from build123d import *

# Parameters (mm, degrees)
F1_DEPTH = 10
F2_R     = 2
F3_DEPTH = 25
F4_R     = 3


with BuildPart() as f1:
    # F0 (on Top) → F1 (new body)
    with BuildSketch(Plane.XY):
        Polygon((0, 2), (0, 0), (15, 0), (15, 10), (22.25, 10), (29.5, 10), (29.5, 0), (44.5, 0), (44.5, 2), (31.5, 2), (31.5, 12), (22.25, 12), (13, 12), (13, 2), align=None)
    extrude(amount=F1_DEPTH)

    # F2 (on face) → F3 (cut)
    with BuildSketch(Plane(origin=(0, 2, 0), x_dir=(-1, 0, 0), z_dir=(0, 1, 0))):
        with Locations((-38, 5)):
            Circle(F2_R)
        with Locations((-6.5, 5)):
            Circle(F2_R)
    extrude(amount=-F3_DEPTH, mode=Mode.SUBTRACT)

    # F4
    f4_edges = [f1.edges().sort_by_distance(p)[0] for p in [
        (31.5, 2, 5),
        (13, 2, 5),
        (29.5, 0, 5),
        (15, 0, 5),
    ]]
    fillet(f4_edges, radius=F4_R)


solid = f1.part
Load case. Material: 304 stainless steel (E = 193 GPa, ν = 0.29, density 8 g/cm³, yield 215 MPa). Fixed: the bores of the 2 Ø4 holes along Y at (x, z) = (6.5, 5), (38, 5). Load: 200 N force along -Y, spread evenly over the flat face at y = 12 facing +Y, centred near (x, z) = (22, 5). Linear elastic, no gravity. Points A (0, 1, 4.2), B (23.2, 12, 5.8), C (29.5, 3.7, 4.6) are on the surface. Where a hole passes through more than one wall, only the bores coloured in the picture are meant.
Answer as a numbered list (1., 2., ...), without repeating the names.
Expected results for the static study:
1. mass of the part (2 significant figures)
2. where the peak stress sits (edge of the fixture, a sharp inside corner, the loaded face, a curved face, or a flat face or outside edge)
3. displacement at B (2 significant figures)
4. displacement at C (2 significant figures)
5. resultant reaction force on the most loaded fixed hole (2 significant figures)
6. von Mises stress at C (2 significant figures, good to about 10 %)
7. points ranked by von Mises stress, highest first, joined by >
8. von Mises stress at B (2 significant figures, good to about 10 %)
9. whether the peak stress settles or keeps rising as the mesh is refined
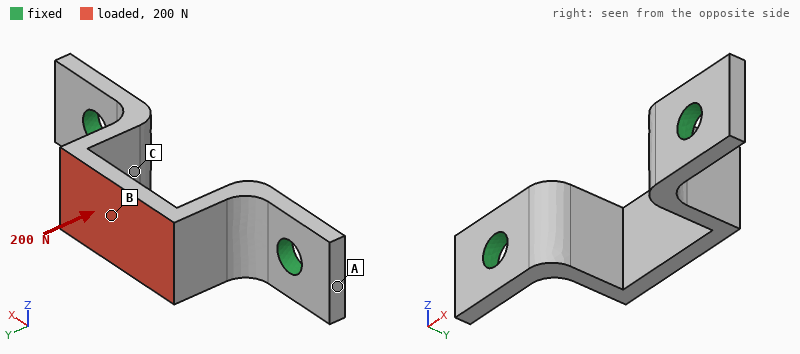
1. 9.9 g
2. edge of the fixture
3. 3.9 µm
4. 2.0 µm
5. 120 N
6. 12 MPa
7. B > C > A
8. 20 MPa
9. keeps rising
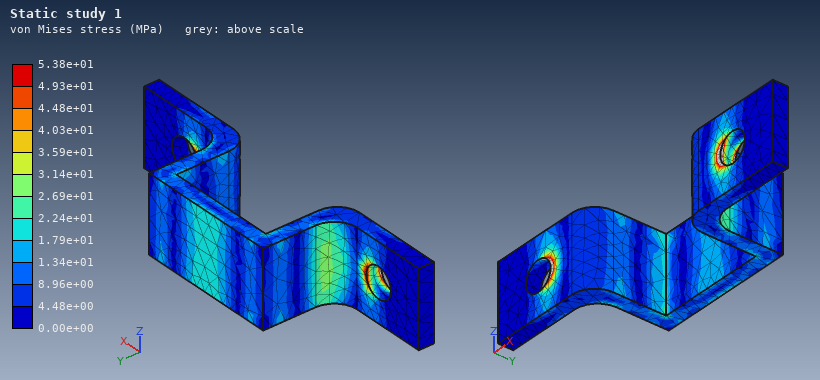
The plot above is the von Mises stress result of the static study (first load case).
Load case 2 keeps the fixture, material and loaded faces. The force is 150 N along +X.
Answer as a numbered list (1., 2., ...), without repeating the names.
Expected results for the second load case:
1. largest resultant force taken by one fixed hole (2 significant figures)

1. 91 N
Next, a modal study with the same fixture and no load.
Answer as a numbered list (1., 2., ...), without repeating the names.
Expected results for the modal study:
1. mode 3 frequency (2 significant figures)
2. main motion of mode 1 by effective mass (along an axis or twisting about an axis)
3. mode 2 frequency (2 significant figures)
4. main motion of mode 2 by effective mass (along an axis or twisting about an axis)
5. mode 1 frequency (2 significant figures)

1. 14 kHz
2. along Z
3. 10 kHz
4. along X
5. 8000 Hz
